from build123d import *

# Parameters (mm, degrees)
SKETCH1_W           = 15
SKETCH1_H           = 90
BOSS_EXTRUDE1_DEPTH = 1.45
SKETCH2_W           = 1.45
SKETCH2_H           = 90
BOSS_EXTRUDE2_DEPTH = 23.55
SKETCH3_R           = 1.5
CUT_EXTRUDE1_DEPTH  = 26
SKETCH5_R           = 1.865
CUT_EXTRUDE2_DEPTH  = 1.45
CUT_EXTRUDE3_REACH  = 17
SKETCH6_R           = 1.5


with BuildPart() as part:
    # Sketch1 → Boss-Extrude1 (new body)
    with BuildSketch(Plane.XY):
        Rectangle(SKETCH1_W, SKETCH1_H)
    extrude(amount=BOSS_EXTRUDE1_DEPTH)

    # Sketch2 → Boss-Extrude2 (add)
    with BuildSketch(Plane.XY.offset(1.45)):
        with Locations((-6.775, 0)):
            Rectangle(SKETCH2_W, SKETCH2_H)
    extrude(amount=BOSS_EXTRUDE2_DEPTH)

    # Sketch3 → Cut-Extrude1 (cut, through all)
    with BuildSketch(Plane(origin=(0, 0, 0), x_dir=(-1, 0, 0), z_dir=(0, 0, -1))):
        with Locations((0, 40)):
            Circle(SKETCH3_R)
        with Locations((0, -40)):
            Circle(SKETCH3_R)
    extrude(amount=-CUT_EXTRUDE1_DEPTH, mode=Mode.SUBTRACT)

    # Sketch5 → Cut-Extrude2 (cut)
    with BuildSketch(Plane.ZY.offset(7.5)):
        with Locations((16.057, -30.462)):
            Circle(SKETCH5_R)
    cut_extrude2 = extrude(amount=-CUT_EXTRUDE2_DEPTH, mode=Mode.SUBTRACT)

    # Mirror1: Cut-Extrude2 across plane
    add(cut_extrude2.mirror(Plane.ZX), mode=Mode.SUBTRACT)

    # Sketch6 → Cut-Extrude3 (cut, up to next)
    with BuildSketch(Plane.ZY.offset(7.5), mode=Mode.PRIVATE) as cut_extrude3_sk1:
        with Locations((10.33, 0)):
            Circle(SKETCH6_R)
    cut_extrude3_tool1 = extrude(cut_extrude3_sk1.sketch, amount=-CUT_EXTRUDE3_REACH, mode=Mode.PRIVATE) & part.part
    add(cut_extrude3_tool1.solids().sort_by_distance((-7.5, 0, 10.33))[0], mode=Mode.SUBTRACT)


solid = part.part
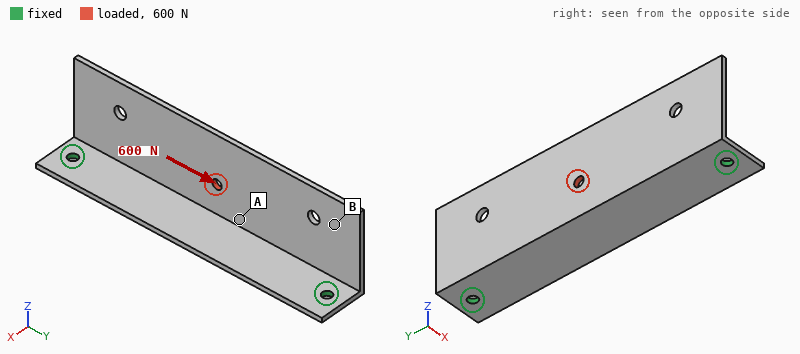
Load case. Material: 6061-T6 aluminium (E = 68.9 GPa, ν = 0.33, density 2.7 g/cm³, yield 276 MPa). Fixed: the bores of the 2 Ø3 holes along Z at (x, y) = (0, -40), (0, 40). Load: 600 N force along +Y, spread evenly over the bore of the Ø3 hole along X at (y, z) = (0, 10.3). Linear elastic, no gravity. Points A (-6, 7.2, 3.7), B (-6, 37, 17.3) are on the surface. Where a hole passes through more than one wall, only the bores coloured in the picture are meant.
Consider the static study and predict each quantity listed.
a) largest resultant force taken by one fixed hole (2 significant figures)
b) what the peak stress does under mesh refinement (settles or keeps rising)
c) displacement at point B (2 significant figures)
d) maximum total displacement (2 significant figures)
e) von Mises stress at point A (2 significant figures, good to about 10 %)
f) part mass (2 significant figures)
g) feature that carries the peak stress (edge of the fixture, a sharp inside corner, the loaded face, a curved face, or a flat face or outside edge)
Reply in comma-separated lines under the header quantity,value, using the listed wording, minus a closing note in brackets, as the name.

quantity,value
largest resultant force taken by one fixed hole,310 N
what the peak stress does under mesh refinement,keeps rising
displacement at point B,52 µm
maximum total displacement,82 µm
von Mises stress at point A,18 MPa
part mass,13 g
feature that carries the peak stress,edge of the fixture
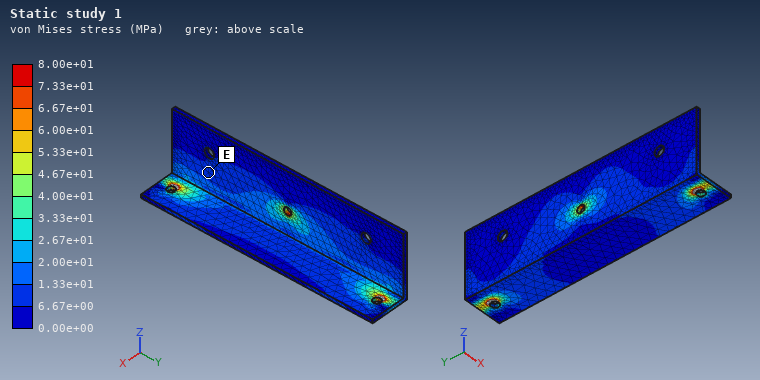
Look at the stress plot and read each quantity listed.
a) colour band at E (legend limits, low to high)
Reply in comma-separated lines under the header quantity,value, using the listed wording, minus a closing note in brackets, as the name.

quantity,value
colour band at E,6.67e+00 to 1.33e+01 MPa
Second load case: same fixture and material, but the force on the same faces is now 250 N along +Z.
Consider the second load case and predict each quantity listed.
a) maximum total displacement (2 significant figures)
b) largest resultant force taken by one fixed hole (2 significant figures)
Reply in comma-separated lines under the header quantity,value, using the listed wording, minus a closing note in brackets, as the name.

quantity,value
maximum total displacement,0.20 mm
largest resultant force taken by one fixed hole,160 N
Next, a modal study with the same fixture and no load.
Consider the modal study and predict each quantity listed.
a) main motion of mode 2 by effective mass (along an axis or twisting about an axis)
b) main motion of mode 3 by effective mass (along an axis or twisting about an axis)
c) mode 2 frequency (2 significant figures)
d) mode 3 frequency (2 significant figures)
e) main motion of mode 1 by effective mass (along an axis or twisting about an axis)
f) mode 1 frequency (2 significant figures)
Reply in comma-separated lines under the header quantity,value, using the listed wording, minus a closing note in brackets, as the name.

quantity,value
main motion of mode 2 by effective mass,twisting about Z
main motion of mode 3 by effective mass,along Z
mode 2 frequency,1800 Hz
mode 3 frequency,2600 Hz
main motion of mode 1 by effective mass,along X
mode 1 frequency,980 Hz
